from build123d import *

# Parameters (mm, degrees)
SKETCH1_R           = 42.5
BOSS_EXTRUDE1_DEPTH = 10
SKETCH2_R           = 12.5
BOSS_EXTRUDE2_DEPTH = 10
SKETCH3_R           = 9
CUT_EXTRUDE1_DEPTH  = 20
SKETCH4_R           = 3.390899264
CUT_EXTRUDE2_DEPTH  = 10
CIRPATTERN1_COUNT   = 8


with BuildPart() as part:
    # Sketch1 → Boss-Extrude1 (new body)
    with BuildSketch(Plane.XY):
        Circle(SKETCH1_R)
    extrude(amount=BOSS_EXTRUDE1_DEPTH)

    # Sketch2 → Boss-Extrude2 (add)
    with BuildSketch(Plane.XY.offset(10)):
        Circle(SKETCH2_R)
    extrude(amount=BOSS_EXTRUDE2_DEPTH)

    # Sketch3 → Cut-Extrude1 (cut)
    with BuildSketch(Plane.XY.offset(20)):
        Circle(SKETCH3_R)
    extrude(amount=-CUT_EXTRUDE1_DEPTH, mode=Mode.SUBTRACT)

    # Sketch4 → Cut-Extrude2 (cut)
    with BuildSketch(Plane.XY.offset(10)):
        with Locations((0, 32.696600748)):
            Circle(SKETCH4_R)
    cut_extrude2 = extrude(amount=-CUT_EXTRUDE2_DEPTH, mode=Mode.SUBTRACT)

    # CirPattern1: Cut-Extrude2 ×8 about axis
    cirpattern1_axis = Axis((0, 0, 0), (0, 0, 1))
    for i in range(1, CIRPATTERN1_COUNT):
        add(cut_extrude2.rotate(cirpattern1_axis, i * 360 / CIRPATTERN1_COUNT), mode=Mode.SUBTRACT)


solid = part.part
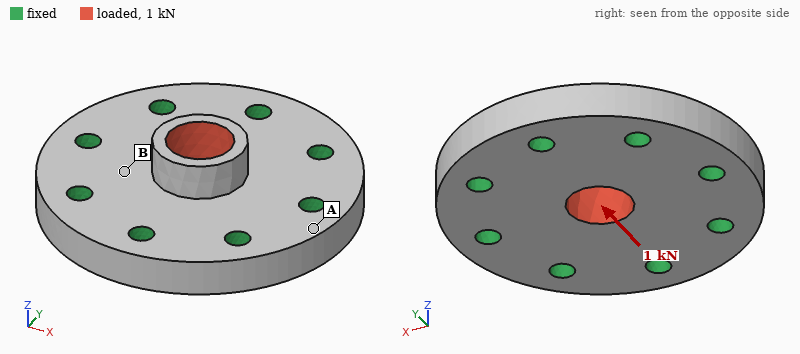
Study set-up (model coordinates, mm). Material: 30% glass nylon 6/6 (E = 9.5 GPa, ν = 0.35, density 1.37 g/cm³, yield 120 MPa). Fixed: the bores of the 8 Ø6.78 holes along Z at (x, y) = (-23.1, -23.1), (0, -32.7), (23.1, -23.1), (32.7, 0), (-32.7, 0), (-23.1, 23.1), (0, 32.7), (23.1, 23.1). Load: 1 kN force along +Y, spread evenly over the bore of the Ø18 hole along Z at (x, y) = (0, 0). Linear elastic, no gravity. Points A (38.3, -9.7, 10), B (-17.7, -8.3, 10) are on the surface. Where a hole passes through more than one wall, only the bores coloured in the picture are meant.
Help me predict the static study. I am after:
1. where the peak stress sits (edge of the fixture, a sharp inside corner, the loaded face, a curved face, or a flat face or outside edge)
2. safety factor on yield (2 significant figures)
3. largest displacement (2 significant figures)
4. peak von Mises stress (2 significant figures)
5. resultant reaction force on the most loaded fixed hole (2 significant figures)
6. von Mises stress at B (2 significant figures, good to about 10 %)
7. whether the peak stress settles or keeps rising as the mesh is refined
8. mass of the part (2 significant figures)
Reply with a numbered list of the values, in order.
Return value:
1. the loaded face
2. 21
3. 16 µm
4. 5.8 MPa
5. 220 N
6. 1.3 MPa
7. settles
8. 74 g
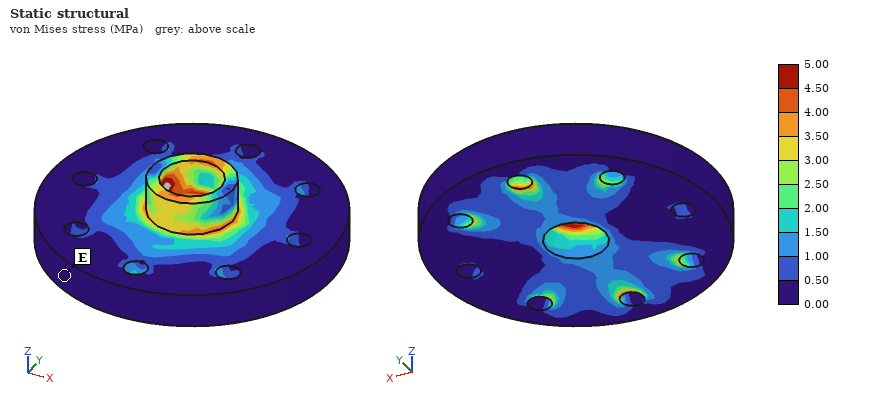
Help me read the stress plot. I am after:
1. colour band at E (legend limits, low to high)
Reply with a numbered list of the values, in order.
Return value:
1. 0.00 to 0.50 MPa
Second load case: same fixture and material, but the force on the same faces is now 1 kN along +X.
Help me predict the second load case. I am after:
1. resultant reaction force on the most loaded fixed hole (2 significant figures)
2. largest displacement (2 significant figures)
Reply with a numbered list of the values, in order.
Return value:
1. 220 N
2. 16 µm
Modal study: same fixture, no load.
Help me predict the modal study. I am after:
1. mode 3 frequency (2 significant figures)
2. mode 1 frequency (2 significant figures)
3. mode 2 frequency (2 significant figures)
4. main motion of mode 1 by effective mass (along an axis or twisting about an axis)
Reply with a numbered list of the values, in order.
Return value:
1. 14 kHz
2. 10 kHz
3. 14 kHz
4. along Z
